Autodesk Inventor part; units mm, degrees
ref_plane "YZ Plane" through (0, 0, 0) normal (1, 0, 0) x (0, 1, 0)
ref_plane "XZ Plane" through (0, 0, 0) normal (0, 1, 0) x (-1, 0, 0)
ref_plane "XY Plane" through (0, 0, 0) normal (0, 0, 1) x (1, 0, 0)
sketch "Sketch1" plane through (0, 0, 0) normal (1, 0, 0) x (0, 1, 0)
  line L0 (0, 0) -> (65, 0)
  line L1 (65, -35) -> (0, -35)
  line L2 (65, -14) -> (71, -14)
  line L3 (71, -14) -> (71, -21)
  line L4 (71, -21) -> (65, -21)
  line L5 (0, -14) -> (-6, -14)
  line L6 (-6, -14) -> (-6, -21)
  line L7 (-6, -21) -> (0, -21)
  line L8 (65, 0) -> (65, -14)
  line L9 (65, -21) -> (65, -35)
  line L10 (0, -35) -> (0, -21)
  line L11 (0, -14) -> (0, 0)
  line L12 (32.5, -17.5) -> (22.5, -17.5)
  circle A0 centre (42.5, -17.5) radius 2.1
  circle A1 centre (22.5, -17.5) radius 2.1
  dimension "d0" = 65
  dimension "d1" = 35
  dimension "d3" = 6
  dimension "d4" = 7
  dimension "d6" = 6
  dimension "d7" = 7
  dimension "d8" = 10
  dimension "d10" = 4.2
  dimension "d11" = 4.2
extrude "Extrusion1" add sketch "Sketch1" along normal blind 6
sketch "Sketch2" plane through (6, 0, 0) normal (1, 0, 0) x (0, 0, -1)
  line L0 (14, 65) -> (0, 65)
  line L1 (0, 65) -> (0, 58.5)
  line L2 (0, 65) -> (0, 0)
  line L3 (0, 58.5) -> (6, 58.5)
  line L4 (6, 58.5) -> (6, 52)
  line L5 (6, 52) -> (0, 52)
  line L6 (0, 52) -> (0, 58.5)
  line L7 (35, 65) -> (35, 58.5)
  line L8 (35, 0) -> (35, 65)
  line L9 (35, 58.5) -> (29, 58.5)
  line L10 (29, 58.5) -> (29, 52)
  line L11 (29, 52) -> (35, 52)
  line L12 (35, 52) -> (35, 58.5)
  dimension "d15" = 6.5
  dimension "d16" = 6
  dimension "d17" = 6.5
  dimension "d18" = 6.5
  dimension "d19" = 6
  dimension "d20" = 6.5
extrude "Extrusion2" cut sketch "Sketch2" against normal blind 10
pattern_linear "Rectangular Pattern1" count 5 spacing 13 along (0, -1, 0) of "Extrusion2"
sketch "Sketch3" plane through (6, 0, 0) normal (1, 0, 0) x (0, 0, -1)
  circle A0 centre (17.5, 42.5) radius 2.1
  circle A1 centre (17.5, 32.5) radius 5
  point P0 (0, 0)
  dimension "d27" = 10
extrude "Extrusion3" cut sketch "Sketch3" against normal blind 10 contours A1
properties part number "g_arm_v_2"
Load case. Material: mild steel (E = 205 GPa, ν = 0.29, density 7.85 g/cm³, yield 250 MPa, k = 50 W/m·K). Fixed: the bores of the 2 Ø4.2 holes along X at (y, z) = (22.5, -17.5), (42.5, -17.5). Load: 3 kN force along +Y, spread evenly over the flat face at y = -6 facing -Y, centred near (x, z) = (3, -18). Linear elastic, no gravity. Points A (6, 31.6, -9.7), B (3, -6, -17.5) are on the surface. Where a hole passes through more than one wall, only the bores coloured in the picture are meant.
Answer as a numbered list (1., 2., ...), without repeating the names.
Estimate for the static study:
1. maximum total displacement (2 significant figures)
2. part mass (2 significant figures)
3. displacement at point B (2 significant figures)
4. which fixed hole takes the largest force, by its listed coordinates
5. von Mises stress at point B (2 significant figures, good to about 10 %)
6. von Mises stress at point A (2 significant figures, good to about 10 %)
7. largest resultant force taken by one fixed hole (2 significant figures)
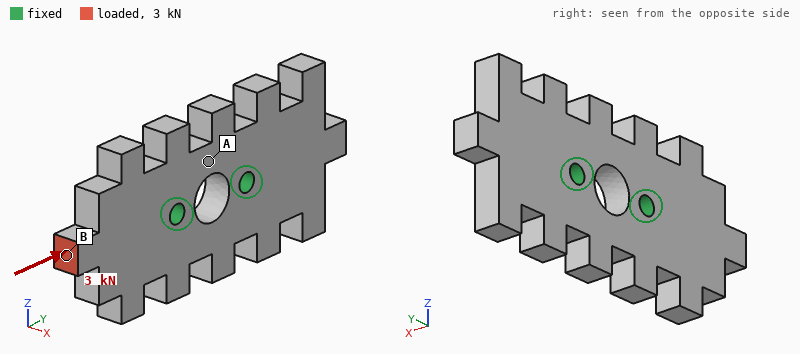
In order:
1. 6.2 µm
2. 88 g
3. 6.1 µm
4. (22.5, -17.5)
5. 73 MPa
6. 10 MPa
7. 2.5 kN
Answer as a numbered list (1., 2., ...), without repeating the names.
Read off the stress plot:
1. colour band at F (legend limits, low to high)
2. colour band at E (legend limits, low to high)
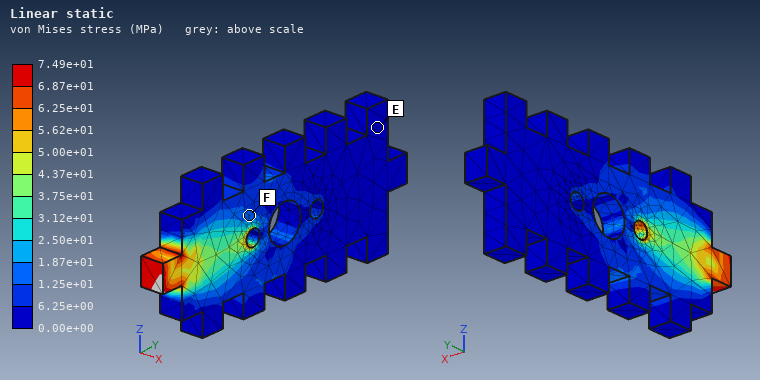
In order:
1. 1.25e+01 to 1.87e+01 MPa
2. 0.00e+00 to 6.25e+00 MPa
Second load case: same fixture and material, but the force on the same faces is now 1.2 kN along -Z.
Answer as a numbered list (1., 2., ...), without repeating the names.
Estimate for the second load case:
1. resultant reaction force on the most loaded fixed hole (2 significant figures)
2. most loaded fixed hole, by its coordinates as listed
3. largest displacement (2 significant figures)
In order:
1. 2.2 kN
2. (22.5, -17.5)
3. 28 µm
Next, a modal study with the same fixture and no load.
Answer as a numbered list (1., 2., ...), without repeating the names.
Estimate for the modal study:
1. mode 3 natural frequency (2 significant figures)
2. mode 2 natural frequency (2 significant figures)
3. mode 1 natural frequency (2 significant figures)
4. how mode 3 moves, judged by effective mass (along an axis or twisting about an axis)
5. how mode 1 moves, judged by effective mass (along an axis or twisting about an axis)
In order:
1. 9700 Hz
2. 7300 Hz
3. 6700 Hz
4. twisting about Y
5. along X
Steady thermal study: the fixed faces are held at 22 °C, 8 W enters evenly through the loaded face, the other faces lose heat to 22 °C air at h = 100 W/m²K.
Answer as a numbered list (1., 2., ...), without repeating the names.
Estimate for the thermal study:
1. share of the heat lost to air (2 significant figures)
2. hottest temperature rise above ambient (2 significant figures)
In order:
1. 34 %
2. 49 K
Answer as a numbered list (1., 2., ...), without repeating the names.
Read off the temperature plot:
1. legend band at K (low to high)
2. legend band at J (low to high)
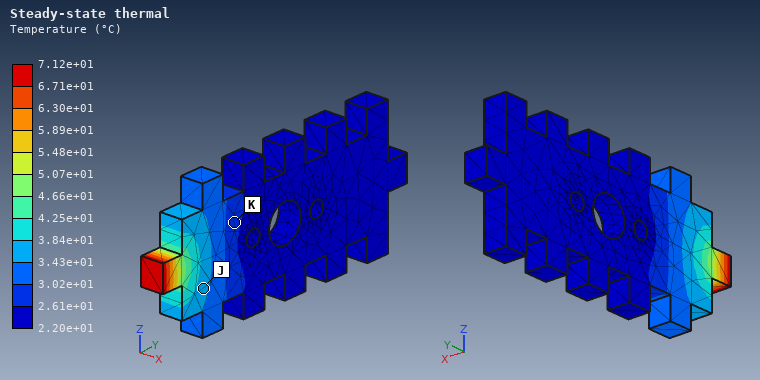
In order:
1. 2.61e+01 to 3.02e+01 °C
2. 3.43e+01 to 3.84e+01 °C
